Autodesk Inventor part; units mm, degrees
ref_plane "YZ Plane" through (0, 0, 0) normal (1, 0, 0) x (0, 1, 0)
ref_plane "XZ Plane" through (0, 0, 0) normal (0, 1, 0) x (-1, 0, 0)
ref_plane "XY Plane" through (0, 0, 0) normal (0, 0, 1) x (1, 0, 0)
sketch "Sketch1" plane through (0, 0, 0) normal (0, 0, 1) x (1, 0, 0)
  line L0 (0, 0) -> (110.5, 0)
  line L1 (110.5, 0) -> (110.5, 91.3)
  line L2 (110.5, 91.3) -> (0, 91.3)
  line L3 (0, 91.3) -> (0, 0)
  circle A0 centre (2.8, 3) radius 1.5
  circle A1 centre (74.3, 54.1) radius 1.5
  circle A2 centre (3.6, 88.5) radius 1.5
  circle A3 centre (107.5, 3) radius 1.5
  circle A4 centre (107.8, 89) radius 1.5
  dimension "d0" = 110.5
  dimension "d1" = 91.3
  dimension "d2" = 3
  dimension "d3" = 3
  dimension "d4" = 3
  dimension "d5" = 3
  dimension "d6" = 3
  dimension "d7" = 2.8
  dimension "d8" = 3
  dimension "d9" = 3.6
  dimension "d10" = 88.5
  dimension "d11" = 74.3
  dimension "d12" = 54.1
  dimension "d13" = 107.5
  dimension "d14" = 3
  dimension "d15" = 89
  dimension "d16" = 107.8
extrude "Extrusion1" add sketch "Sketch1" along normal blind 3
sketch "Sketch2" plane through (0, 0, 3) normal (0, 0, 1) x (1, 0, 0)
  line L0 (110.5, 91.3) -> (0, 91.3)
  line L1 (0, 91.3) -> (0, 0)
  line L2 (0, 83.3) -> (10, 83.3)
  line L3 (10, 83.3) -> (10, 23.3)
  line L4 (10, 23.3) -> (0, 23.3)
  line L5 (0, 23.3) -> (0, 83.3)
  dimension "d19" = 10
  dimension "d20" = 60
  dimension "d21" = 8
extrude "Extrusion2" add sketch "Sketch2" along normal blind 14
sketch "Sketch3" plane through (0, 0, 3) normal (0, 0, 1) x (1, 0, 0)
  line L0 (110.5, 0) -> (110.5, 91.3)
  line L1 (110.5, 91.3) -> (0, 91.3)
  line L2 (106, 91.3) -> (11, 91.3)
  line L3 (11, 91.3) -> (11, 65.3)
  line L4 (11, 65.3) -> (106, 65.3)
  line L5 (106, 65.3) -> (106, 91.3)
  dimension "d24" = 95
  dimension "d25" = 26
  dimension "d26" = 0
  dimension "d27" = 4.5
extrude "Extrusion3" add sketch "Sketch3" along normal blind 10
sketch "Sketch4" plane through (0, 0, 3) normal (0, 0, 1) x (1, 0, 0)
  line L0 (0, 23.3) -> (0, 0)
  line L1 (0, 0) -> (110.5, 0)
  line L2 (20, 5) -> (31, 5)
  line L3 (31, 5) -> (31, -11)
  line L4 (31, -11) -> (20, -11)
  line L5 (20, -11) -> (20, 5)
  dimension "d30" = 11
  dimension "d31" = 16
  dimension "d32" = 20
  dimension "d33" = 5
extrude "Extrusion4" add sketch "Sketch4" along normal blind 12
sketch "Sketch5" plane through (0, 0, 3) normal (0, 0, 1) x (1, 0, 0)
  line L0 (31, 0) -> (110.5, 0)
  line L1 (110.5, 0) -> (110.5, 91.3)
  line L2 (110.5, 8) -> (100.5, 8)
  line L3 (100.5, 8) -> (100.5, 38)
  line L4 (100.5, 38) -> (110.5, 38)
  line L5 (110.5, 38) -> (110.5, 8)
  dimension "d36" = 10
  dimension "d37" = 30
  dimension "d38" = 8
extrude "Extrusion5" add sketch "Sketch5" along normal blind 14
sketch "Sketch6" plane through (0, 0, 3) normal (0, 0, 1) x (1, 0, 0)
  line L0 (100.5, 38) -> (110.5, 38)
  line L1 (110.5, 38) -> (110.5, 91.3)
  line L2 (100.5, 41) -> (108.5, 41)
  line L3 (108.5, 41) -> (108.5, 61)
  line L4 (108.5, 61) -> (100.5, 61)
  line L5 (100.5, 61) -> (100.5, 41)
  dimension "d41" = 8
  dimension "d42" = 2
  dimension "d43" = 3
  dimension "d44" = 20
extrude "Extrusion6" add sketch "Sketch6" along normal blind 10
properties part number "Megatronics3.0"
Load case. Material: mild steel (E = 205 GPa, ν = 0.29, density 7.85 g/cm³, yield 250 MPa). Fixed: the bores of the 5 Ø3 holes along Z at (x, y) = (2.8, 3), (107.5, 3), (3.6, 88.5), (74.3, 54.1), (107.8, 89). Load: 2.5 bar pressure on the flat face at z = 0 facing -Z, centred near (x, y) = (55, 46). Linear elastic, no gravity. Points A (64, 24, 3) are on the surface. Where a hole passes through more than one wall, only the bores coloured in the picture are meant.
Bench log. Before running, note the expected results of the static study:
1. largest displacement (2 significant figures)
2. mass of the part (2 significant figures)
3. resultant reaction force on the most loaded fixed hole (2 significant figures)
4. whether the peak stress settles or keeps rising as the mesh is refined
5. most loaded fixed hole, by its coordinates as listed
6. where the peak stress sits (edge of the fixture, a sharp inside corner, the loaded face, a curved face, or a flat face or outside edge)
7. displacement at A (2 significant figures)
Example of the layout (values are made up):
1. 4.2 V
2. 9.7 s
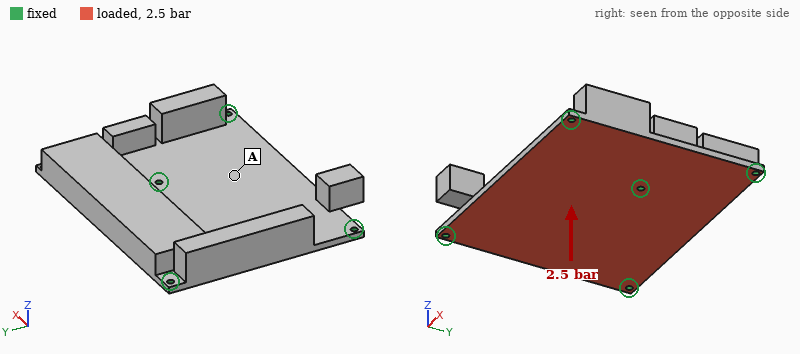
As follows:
1. 0.14 mm
2. 560 g
3. 1.2 kN
4. keeps rising
5. (74.3, 54.1)
6. edge of the fixture
7. 0.081 mm
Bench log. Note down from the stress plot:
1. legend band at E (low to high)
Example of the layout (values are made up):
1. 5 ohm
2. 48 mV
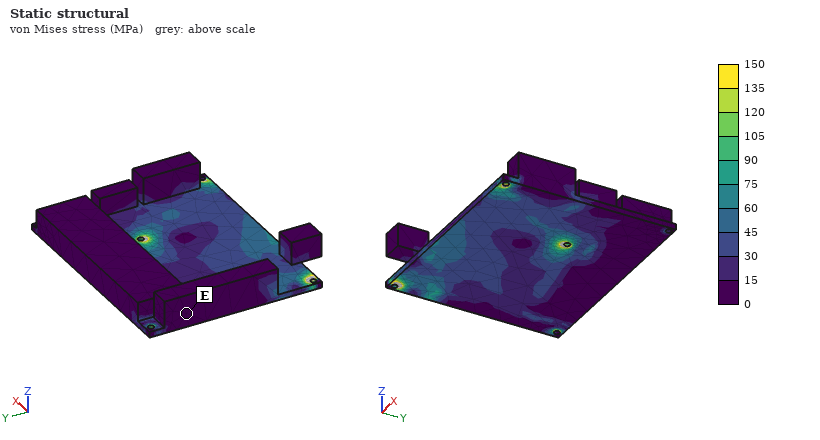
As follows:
1. 0 to 15 MPa
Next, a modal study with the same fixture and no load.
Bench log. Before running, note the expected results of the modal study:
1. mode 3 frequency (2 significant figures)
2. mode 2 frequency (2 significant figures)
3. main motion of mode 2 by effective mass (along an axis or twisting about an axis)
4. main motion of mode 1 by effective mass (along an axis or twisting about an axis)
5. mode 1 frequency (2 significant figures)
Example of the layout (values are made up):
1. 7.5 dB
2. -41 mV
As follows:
1. 3000 Hz
2. 2500 Hz
3. along Z
4. along Z
5. 1600 Hz
